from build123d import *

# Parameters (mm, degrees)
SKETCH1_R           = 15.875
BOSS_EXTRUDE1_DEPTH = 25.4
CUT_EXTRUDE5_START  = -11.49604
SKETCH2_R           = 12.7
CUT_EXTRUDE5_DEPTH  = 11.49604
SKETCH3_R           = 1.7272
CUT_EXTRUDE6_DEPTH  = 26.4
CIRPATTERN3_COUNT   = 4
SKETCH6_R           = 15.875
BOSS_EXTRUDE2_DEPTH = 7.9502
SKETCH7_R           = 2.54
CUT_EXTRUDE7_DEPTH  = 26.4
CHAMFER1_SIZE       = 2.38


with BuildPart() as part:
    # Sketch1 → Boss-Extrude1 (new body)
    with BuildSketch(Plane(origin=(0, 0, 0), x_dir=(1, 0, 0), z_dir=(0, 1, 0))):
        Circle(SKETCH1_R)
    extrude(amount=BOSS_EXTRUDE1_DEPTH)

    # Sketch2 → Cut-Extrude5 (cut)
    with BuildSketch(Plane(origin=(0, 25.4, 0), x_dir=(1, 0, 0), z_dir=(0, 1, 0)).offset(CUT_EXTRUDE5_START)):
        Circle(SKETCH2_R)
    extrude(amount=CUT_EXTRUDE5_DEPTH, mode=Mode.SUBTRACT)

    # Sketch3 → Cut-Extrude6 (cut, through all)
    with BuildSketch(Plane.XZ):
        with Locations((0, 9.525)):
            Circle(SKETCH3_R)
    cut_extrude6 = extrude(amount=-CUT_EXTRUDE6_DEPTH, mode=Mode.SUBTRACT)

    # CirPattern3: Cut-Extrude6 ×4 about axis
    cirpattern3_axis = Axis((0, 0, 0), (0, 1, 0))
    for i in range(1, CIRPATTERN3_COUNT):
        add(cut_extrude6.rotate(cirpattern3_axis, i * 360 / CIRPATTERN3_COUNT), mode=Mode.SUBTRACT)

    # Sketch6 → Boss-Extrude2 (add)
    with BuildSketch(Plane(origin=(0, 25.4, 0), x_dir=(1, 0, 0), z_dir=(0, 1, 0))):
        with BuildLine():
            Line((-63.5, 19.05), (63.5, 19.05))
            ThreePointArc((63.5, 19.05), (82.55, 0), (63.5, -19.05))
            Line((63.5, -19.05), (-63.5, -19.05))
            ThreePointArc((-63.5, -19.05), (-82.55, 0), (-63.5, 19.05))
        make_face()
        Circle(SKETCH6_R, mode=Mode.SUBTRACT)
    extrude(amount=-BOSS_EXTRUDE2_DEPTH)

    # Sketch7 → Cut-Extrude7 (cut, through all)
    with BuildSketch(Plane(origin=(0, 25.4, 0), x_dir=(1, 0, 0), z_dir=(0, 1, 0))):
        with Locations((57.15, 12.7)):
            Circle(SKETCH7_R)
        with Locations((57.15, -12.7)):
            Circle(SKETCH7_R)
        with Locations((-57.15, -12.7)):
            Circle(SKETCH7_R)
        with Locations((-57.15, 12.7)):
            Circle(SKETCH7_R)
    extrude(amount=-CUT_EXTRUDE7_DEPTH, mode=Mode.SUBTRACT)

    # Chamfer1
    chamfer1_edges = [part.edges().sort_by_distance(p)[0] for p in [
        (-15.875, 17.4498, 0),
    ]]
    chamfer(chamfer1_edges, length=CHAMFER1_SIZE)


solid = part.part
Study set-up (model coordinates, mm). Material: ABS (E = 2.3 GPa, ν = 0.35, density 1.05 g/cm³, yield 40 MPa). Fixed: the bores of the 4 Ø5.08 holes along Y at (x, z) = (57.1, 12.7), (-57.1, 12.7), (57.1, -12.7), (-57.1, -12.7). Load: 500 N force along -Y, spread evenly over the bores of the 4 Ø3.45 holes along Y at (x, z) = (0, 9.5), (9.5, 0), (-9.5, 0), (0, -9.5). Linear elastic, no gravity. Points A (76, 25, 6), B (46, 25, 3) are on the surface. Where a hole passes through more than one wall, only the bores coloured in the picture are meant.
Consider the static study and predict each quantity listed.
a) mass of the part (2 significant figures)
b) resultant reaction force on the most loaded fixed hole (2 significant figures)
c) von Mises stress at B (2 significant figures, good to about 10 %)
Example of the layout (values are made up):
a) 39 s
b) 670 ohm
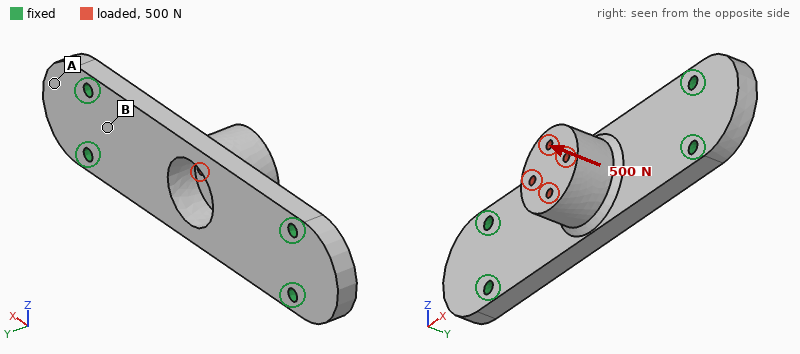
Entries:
a) 57 g
b) 180 N
c) 7.6 MPa
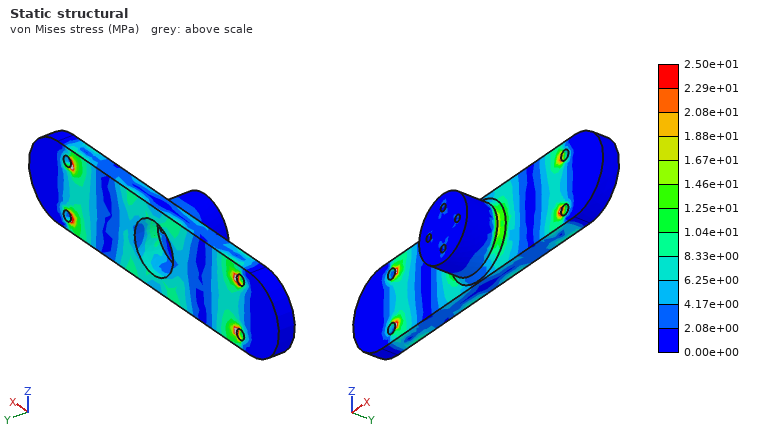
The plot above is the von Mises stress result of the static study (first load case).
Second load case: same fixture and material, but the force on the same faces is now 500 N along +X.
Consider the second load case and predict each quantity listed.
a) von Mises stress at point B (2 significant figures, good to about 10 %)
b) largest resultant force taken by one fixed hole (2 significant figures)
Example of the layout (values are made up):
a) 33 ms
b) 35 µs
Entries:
a) 1.8 MPa
b) 130 N
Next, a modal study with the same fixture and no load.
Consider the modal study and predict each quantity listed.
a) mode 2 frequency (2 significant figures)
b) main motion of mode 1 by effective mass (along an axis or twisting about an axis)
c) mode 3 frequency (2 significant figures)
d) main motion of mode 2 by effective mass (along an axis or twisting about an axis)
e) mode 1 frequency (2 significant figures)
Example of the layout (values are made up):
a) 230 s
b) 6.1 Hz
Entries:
a) 1100 Hz
b) along Y
c) 1900 Hz
d) along Z
e) 850 Hz
